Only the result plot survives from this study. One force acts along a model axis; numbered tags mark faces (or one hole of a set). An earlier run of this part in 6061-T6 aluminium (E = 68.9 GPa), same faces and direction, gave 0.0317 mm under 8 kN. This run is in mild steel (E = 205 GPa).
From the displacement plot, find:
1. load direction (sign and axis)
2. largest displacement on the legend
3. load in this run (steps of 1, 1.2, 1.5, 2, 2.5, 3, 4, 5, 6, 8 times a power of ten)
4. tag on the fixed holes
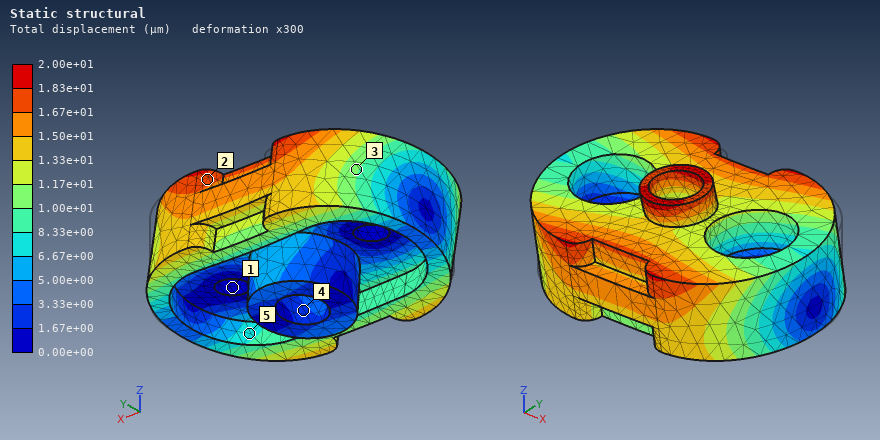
-Y
2.00e+01 µm
15 kN
1
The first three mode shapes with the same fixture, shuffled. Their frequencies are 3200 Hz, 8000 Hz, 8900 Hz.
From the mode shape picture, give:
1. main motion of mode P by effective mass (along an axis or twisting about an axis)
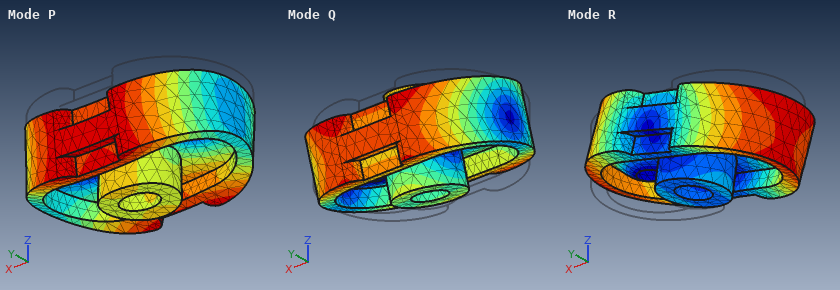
along Z
